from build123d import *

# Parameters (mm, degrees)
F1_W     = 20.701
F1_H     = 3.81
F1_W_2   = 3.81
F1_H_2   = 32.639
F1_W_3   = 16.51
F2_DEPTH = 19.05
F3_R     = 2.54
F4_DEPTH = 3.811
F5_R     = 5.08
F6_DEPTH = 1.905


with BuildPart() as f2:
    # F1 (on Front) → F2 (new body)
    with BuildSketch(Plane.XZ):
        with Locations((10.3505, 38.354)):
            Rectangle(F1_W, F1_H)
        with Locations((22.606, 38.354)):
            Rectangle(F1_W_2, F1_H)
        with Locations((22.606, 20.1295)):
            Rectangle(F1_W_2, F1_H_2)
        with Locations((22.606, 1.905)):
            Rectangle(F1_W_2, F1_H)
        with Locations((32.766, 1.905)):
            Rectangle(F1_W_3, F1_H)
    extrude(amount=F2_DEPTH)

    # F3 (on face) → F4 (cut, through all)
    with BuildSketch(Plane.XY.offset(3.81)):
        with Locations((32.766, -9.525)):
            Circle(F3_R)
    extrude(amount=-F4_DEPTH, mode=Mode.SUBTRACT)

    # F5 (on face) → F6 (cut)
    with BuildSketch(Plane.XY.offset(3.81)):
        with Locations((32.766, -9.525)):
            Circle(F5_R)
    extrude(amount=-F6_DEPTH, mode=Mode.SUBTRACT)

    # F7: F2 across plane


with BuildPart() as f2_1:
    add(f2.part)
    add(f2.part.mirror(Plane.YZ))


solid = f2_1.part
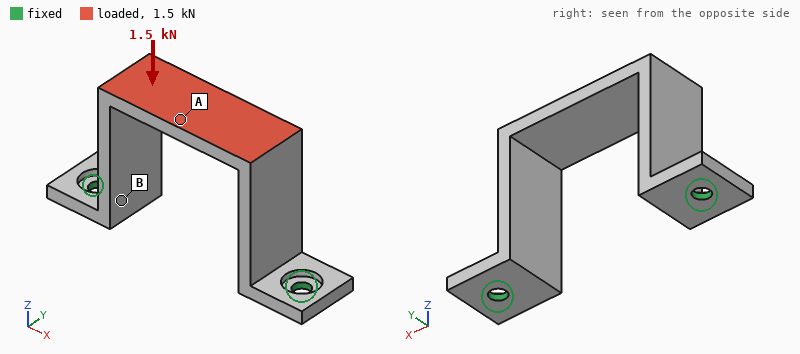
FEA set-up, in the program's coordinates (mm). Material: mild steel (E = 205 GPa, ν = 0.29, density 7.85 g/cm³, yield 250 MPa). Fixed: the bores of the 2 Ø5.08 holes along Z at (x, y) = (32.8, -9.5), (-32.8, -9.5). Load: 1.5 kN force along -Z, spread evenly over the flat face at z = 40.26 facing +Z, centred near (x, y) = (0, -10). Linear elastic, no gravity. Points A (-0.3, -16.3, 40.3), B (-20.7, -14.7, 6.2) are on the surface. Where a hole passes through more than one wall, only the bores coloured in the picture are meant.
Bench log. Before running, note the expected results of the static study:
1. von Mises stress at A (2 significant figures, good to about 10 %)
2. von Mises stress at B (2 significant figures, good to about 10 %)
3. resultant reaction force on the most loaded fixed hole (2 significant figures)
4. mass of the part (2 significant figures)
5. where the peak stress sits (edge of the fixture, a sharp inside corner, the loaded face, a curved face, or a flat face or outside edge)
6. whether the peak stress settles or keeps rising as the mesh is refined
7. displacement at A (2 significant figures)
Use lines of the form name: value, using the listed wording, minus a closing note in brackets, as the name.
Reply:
von Mises stress at A: 78 MPa
von Mises stress at B: 45 MPa
resultant reaction force on the most loaded fixed hole: 780 N
mass of the part: 85 g
where the peak stress sits: edge of the fixture
whether the peak stress settles or keeps rising as the mesh is refined: keeps rising
displacement at A: 47 µm
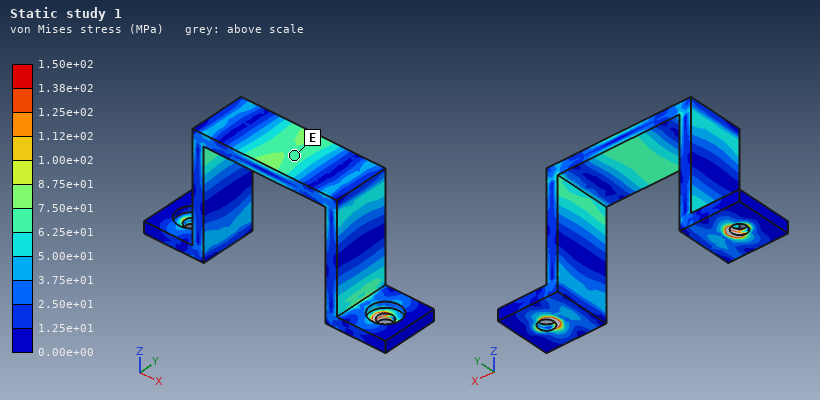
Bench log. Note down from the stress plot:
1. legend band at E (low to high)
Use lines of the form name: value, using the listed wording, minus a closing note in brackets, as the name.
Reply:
legend band at E: 6.25e+01 to 7.50e+01 MPa
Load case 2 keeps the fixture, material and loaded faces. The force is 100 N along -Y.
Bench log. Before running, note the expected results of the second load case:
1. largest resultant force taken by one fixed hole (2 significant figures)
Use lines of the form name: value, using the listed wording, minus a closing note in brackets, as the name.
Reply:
largest resultant force taken by one fixed hole: 50 N
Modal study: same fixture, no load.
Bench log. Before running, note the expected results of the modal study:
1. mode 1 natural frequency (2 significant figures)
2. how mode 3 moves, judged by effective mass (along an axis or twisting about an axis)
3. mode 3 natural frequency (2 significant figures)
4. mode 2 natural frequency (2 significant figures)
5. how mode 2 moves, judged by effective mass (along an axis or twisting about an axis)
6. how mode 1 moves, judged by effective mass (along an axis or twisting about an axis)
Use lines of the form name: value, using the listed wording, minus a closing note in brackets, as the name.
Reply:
mode 1 natural frequency: 1200 Hz
how mode 3 moves, judged by effective mass: twisting about Z
mode 3 natural frequency: 2600 Hz
mode 2 natural frequency: 1600 Hz
how mode 2 moves, judged by effective mass: along X
how mode 1 moves, judged by effective mass: along Y
